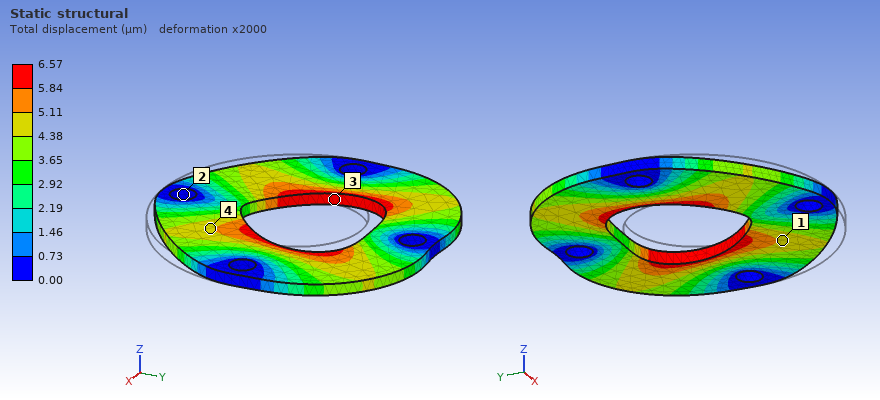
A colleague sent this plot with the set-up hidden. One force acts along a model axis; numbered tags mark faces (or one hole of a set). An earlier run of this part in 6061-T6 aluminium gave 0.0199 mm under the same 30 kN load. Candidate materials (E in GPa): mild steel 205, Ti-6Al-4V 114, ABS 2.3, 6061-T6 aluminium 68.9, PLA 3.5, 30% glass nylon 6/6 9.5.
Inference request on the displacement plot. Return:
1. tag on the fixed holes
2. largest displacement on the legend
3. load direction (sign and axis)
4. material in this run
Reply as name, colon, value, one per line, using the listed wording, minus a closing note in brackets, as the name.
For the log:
tag on the fixed holes: 2
largest displacement on the legend: 6.57 µm
load direction: +Y
material in this run: mild steel
